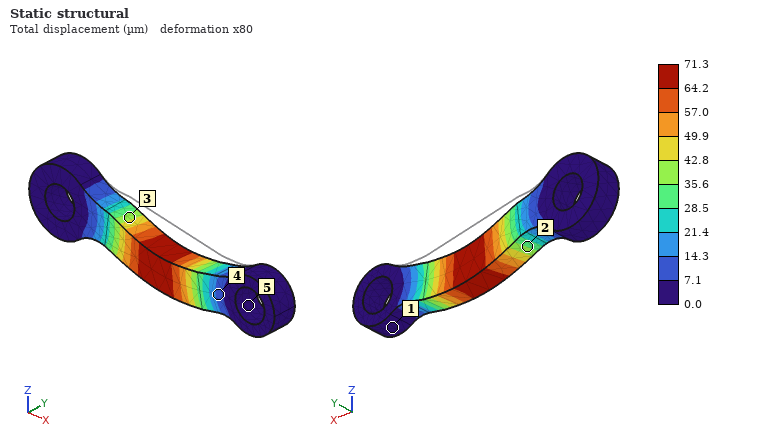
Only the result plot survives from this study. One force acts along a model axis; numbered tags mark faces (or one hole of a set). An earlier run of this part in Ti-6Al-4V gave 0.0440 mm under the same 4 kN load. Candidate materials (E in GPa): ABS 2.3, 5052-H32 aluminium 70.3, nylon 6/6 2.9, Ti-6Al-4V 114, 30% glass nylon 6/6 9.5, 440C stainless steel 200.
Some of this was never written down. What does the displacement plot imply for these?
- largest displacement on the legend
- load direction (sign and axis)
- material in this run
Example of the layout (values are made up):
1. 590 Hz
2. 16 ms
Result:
1. 71.3 µm
2. -Z
3. 5052-H32 aluminium
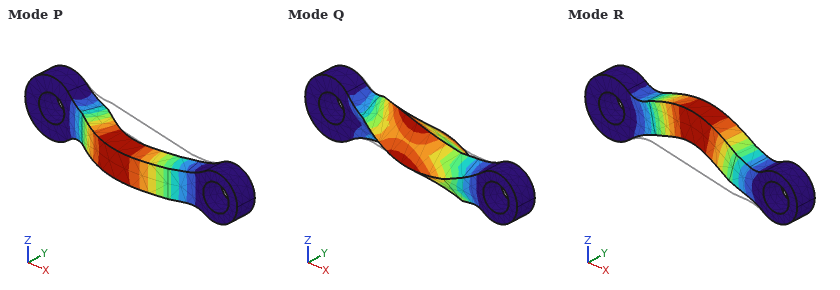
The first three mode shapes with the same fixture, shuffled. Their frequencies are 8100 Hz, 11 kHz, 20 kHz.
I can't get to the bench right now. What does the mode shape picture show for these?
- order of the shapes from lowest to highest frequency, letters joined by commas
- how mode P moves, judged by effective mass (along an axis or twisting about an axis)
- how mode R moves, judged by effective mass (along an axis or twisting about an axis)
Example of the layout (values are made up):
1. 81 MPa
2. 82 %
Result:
1. P, R, Q
2. along Y
3. along Z
